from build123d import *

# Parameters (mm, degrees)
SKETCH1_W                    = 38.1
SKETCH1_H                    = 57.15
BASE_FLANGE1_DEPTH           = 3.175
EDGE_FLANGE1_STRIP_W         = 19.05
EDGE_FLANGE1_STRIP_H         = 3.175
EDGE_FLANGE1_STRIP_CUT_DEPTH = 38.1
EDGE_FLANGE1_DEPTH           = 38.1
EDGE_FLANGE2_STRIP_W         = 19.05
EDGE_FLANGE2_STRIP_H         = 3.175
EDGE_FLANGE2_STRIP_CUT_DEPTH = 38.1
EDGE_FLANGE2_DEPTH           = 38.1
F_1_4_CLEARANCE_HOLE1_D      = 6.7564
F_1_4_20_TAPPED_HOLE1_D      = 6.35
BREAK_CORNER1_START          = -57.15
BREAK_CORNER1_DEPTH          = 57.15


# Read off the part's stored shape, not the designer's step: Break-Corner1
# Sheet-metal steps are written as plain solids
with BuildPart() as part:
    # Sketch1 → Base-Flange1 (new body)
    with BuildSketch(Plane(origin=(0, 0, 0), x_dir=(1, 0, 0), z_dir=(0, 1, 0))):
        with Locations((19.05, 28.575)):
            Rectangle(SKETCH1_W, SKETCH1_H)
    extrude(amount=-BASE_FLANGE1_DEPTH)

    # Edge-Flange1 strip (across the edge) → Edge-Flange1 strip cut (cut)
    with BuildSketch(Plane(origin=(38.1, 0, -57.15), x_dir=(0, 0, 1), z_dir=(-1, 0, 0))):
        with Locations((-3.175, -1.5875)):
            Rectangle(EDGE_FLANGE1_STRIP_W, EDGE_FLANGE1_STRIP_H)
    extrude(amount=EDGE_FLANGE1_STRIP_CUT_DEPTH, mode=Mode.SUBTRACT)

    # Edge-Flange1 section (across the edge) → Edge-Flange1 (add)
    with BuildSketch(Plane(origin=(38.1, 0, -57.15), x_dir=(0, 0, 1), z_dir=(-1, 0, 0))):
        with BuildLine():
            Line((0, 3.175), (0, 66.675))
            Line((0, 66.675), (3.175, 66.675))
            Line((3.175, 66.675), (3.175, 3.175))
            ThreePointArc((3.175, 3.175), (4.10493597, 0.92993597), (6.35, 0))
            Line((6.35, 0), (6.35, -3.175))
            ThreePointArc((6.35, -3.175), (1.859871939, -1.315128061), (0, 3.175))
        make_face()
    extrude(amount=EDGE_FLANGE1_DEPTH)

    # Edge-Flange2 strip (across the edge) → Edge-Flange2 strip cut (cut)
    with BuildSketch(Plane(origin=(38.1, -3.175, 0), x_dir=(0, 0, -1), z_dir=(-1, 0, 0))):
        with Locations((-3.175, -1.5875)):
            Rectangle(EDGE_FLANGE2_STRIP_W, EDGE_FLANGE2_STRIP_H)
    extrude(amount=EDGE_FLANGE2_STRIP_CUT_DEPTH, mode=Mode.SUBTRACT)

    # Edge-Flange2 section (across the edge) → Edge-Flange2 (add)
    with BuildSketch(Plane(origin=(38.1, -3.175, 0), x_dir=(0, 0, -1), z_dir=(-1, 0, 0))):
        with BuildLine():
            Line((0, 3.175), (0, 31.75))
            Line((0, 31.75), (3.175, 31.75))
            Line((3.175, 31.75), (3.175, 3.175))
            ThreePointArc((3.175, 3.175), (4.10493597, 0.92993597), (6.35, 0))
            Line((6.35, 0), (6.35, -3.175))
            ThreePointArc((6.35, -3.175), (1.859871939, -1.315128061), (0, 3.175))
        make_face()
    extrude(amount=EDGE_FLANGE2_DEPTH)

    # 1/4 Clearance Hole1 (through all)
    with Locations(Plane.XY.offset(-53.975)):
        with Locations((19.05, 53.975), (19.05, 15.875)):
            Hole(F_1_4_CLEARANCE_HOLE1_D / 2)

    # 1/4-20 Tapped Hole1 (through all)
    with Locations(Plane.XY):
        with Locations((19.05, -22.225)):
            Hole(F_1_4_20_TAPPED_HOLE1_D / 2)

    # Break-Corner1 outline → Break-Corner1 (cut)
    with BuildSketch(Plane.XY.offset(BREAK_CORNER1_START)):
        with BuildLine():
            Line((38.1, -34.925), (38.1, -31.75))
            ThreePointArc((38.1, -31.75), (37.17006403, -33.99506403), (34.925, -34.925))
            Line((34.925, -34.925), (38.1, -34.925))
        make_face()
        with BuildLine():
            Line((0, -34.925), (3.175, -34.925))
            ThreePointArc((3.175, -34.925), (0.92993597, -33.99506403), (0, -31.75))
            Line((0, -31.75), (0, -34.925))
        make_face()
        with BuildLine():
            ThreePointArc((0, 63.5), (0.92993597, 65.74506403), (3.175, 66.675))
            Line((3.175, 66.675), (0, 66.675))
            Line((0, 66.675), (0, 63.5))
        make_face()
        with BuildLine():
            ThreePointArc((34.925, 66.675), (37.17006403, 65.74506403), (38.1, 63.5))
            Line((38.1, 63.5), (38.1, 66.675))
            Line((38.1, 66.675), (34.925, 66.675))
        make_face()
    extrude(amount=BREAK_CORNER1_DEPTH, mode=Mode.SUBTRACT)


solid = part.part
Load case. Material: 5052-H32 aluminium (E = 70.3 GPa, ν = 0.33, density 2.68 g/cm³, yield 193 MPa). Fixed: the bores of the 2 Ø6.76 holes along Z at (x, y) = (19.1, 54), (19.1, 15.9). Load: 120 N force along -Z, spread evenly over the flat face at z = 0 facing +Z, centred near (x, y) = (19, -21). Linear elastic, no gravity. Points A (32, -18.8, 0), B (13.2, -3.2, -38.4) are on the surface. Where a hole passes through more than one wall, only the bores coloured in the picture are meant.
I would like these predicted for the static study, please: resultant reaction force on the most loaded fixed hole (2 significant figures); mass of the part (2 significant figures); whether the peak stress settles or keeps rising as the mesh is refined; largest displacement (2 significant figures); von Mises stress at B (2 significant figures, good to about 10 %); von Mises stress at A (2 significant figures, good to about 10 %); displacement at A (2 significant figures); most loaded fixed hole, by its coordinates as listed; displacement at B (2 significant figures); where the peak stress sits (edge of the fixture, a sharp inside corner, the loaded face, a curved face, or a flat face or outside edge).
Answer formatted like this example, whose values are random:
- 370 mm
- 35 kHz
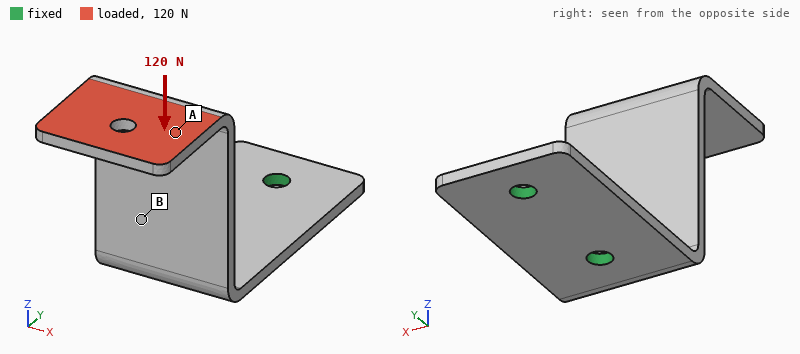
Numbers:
- 140 N
- 48 g
- keeps rising
- 1.2 mm
- 34 MPa
- 8.8 MPa
- 0.98 mm
- (19.1, 15.9)
- 0.19 mm
- edge of the fixture
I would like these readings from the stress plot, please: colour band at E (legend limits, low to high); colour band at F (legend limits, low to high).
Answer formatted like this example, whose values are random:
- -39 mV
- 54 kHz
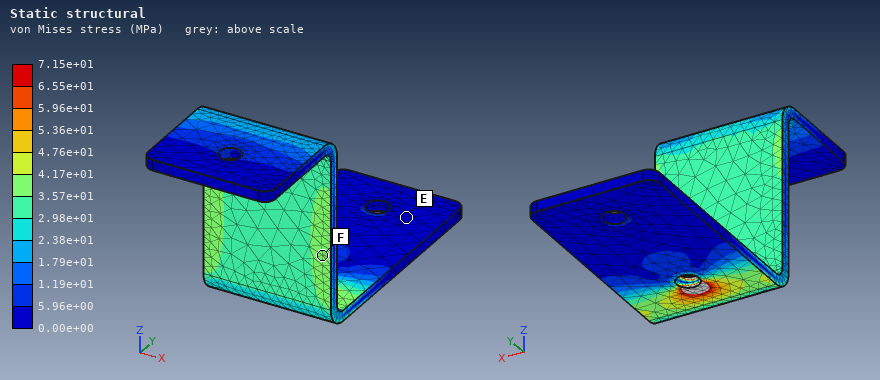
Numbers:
- 0.00e+00 to 5.96e+00 MPa
- 3.57e+01 to 4.17e+01 MPa
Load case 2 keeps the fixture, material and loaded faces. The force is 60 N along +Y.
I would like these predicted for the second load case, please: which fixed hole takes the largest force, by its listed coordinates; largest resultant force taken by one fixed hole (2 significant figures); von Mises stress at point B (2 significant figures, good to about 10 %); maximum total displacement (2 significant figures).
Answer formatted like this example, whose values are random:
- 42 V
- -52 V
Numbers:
- (19.1, 15.9)
- 57 N
- 32 MPa
- 1.1 mm
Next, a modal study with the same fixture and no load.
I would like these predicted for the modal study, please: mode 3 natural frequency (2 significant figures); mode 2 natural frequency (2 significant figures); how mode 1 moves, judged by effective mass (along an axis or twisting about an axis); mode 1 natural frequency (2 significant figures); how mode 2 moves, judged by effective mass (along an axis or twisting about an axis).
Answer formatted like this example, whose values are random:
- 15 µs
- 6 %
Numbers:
- 1200 Hz
- 660 Hz
- along Y
- 330 Hz
- along X
